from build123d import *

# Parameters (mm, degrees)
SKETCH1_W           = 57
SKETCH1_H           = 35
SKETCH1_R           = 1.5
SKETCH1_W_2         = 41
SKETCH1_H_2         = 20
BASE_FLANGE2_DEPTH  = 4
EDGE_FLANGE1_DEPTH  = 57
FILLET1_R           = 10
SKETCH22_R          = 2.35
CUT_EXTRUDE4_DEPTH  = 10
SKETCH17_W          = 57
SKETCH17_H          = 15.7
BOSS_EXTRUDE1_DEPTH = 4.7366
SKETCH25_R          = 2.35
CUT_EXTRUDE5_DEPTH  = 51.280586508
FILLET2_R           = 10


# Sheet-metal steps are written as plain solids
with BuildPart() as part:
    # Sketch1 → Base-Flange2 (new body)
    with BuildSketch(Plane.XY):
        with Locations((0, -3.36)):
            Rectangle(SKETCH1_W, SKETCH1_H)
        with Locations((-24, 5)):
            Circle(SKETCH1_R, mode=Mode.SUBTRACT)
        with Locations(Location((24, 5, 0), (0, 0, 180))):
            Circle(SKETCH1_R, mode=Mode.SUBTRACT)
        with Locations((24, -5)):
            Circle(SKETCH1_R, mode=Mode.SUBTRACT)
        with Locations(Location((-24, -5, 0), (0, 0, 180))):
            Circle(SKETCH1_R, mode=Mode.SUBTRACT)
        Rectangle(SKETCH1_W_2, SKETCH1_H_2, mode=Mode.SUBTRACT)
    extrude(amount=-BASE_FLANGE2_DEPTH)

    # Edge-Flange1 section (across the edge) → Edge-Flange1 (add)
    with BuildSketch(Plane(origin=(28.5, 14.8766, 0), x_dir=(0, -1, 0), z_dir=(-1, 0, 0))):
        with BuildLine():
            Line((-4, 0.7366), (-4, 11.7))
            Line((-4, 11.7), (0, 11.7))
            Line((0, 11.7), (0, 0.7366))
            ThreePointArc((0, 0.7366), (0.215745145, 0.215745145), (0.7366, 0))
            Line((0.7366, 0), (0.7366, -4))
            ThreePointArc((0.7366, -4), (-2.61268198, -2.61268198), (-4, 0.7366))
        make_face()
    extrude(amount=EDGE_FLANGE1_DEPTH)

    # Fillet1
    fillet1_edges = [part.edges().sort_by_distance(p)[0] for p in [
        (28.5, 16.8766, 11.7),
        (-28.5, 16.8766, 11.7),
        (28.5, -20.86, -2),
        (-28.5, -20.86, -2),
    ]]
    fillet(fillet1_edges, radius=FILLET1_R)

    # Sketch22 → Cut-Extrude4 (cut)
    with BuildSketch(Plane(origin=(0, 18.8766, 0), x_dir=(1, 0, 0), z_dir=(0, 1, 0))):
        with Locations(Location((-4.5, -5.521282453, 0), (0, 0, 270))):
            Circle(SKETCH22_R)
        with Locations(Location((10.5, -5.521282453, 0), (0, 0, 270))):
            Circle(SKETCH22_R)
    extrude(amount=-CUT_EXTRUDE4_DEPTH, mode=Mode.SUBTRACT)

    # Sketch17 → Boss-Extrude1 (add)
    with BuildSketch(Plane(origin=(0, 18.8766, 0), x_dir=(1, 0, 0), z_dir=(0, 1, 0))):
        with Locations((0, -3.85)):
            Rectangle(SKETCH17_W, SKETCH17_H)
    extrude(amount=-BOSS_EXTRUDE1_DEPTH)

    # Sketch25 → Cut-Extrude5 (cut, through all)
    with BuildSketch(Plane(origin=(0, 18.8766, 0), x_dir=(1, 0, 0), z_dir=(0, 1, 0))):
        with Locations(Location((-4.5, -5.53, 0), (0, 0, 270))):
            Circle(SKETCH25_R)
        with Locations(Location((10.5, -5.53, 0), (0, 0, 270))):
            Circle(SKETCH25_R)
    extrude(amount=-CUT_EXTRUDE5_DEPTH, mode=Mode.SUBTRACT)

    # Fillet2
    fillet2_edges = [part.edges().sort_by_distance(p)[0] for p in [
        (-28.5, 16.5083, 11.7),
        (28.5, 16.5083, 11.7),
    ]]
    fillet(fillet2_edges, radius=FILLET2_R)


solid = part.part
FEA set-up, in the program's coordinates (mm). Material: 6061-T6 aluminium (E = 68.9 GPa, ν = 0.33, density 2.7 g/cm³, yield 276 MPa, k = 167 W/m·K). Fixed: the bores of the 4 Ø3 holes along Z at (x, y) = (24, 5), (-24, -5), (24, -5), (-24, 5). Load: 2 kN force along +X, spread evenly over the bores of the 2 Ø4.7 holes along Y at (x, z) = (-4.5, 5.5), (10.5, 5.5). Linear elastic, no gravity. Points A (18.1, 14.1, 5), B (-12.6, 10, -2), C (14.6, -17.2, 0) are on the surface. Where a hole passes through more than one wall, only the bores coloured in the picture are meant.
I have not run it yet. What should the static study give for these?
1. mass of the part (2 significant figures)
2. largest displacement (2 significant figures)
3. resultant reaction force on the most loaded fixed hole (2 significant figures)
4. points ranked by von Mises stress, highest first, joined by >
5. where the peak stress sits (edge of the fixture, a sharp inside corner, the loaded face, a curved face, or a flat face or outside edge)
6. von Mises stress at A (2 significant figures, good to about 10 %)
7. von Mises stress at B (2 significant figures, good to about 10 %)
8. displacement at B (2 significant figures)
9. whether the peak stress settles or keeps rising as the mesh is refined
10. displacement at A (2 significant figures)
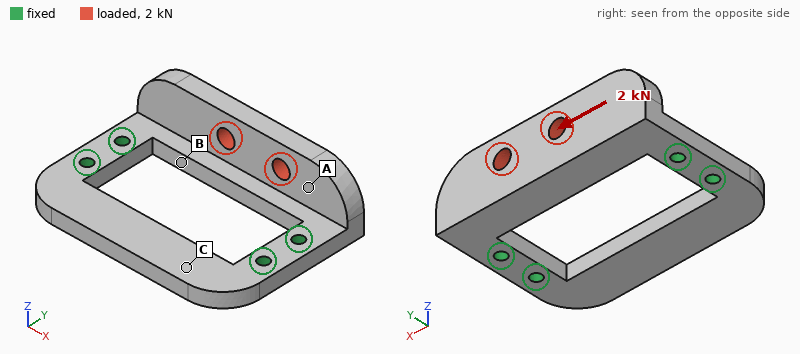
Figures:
22 g
49 µm
1.2 kN
B > A > C
edge of the fixture
33 MPa
48 MPa
24 µm
keeps rising
36 µm
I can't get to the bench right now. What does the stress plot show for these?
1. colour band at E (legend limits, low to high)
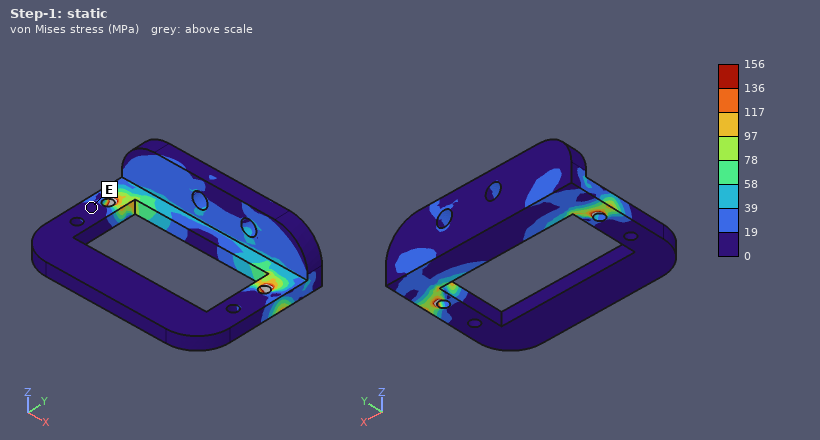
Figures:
0 to 19 MPa
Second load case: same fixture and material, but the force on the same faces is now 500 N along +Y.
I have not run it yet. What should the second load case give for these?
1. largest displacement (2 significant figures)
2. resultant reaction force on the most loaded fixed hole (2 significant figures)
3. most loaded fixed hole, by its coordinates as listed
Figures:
0.13 mm
350 N
(24, 5)
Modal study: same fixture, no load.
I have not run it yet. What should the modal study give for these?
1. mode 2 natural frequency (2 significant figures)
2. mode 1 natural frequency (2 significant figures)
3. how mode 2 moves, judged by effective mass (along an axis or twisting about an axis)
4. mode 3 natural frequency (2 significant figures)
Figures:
5200 Hz
3800 Hz
along Z
8800 Hz
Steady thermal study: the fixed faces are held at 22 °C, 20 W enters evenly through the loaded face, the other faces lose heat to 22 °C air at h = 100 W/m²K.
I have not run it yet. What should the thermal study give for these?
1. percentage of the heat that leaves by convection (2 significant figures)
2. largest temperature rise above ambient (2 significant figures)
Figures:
23 %
24 K
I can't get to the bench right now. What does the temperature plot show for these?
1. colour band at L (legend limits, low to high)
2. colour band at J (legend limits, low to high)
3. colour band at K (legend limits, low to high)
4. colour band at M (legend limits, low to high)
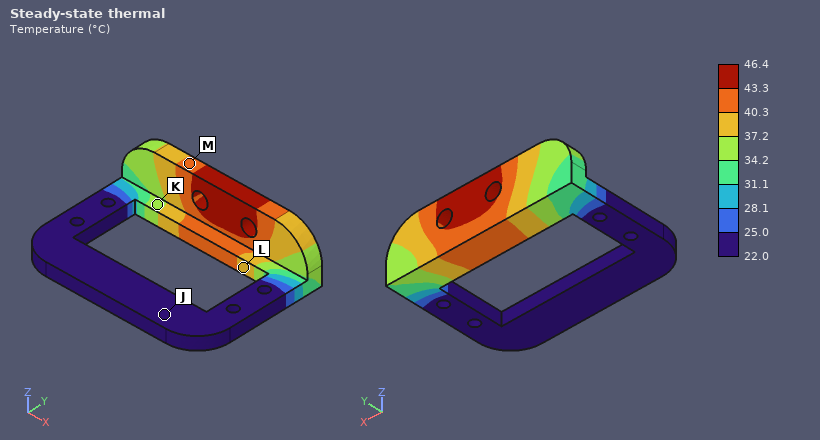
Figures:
37.2 to 40.3 °C
22.0 to 25.0 °C
34.2 to 37.2 °C
40.3 to 43.3 °C
